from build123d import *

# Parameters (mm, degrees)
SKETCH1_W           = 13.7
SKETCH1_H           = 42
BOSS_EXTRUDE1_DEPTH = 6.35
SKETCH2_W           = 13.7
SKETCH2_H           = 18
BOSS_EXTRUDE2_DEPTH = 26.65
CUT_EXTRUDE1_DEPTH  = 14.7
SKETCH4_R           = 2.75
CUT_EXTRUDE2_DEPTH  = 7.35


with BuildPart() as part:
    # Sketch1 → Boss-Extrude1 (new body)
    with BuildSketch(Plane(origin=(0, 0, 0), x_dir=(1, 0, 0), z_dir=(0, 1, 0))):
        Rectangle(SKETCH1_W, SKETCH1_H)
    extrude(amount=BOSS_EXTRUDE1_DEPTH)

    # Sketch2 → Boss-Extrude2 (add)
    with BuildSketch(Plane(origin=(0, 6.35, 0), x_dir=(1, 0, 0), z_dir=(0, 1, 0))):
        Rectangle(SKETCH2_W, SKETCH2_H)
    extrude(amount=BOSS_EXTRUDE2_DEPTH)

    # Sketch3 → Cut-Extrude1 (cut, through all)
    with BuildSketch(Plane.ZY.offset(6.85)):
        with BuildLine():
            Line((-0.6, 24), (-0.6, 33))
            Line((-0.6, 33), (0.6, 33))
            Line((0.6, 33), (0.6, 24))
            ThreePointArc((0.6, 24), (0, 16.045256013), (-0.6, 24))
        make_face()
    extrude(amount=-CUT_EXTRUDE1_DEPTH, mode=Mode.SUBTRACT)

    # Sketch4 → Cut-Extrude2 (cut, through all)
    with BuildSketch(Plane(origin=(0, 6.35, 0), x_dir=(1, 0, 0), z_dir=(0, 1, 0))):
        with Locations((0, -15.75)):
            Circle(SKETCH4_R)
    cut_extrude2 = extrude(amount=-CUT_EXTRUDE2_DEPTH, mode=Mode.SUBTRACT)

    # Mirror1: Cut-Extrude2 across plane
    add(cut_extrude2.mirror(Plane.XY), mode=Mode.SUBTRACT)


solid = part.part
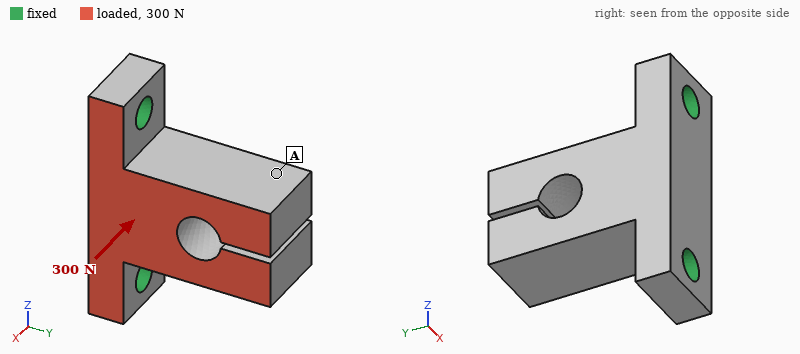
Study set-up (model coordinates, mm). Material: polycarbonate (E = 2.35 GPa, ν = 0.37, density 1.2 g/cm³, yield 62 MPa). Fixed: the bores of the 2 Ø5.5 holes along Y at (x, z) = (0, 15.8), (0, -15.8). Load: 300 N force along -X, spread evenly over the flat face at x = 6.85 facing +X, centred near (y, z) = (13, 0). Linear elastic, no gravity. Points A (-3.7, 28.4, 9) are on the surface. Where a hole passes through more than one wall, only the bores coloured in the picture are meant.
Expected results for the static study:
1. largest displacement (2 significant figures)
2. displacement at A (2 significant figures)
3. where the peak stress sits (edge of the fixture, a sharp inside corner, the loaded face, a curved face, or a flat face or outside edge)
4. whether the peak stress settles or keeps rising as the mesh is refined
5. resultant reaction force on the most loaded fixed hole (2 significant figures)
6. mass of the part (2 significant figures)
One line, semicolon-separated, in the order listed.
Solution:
0.49 mm; 0.40 mm; edge of the fixture; keeps rising; 150 N; 11 g
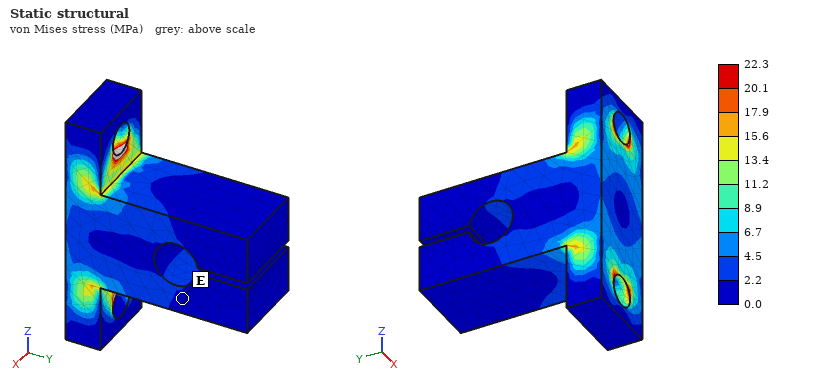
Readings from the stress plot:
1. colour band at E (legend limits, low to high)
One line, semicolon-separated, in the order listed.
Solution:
0.0 to 2.2 MPa
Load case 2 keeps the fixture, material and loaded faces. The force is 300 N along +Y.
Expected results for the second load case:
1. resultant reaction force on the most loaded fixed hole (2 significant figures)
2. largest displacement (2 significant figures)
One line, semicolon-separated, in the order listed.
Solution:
160 N; 0.28 mm
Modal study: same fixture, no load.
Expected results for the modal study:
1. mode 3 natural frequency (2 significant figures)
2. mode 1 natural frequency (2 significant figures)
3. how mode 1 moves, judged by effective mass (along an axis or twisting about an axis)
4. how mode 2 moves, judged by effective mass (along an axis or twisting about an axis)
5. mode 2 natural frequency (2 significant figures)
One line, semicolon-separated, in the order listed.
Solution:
2600 Hz; 1400 Hz; along X; along Z; 2200 Hz
